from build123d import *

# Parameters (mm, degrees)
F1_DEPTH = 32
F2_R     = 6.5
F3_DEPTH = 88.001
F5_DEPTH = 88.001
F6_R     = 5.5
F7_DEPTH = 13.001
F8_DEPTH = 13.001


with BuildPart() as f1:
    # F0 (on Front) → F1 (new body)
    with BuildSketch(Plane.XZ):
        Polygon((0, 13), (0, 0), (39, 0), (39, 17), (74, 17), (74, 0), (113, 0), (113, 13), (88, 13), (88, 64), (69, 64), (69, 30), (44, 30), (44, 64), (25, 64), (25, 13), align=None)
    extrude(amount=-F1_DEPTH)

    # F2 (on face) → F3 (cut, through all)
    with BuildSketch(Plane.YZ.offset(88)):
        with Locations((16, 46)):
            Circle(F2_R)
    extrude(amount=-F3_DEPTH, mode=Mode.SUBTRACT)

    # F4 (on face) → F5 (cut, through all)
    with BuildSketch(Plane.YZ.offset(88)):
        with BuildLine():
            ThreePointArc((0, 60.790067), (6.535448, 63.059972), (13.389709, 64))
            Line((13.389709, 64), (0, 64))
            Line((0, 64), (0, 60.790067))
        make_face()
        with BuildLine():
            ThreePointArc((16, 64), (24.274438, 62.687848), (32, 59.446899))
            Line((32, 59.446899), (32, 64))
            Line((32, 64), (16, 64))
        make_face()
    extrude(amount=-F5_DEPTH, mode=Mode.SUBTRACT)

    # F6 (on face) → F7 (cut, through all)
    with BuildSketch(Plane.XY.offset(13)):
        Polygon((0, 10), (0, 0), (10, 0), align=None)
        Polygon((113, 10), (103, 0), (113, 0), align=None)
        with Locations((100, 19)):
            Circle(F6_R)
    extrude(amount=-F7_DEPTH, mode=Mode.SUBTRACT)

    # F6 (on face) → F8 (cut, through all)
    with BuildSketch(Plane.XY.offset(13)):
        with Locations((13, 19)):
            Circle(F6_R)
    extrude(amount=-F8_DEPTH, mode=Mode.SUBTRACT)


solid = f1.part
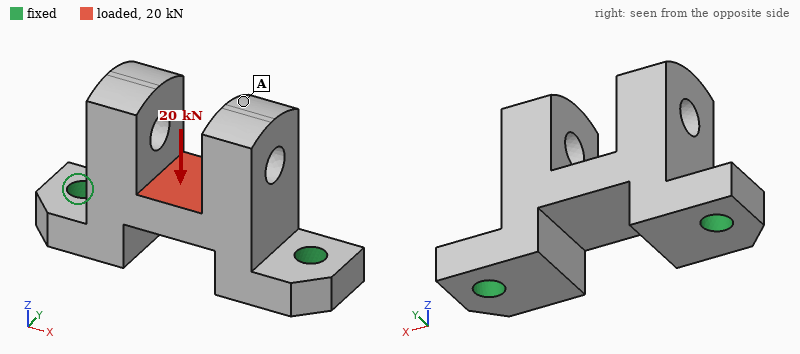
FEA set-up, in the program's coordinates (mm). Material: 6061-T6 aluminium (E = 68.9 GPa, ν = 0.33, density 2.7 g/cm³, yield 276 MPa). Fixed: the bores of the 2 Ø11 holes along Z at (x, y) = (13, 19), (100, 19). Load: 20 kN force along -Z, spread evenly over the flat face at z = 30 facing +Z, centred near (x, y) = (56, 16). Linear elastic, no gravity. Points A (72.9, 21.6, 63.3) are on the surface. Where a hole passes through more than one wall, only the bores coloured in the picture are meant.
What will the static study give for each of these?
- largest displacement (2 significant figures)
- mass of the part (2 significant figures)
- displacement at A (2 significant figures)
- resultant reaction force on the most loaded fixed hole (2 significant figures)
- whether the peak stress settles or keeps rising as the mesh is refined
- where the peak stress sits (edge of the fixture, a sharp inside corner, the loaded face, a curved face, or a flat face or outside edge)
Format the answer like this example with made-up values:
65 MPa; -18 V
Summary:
0.10 mm; 250 g; 0.096 mm; 15 kN; keeps rising; edge of the fixture
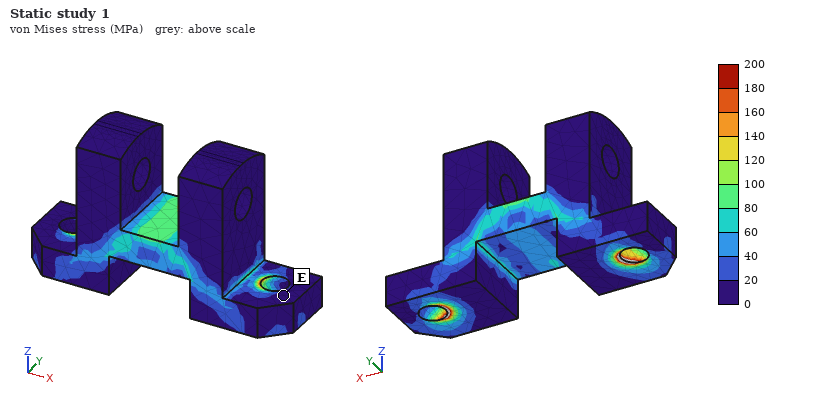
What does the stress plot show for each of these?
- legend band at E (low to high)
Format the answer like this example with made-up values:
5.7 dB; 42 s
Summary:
0 to 20 MPa
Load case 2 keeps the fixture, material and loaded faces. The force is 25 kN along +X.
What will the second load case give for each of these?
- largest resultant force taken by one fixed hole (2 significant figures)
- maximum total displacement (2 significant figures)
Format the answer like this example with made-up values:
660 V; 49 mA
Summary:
15 kN; 65 µm
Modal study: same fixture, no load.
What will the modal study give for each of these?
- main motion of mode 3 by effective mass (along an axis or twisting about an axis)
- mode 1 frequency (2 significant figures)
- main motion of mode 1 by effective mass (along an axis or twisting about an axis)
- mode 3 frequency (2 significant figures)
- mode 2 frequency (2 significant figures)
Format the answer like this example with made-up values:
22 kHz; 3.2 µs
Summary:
along X; 2800 Hz; along Y; 5700 Hz; 4600 Hz
